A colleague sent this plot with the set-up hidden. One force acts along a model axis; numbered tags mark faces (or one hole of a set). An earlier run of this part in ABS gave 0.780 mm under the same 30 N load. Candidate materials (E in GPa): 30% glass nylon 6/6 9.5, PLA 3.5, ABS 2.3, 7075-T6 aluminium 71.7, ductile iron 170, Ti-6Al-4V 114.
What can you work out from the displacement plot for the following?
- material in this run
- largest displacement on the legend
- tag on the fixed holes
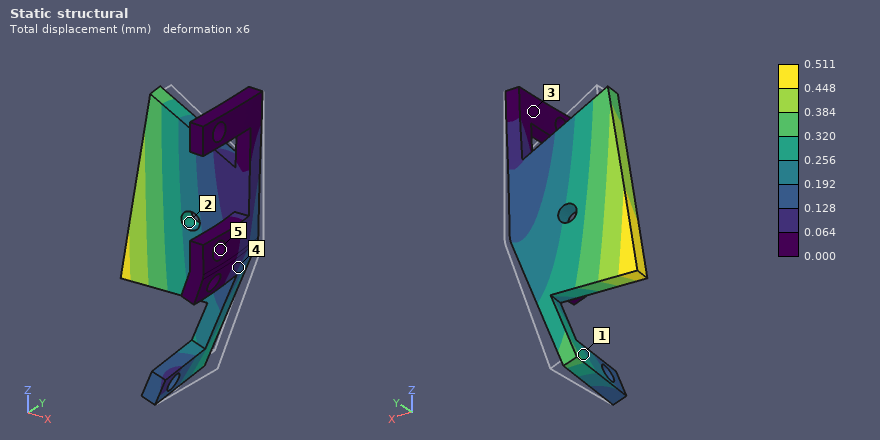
PLA
0.511 mm
5
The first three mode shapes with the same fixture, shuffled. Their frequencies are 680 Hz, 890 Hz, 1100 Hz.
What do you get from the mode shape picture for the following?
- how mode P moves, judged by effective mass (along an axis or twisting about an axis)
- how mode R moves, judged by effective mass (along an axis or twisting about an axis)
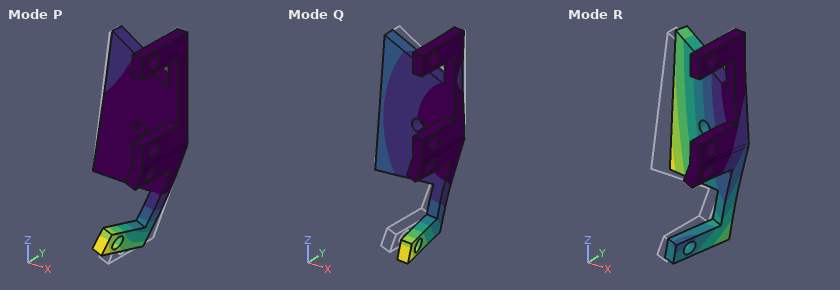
twisting about X
along Y
